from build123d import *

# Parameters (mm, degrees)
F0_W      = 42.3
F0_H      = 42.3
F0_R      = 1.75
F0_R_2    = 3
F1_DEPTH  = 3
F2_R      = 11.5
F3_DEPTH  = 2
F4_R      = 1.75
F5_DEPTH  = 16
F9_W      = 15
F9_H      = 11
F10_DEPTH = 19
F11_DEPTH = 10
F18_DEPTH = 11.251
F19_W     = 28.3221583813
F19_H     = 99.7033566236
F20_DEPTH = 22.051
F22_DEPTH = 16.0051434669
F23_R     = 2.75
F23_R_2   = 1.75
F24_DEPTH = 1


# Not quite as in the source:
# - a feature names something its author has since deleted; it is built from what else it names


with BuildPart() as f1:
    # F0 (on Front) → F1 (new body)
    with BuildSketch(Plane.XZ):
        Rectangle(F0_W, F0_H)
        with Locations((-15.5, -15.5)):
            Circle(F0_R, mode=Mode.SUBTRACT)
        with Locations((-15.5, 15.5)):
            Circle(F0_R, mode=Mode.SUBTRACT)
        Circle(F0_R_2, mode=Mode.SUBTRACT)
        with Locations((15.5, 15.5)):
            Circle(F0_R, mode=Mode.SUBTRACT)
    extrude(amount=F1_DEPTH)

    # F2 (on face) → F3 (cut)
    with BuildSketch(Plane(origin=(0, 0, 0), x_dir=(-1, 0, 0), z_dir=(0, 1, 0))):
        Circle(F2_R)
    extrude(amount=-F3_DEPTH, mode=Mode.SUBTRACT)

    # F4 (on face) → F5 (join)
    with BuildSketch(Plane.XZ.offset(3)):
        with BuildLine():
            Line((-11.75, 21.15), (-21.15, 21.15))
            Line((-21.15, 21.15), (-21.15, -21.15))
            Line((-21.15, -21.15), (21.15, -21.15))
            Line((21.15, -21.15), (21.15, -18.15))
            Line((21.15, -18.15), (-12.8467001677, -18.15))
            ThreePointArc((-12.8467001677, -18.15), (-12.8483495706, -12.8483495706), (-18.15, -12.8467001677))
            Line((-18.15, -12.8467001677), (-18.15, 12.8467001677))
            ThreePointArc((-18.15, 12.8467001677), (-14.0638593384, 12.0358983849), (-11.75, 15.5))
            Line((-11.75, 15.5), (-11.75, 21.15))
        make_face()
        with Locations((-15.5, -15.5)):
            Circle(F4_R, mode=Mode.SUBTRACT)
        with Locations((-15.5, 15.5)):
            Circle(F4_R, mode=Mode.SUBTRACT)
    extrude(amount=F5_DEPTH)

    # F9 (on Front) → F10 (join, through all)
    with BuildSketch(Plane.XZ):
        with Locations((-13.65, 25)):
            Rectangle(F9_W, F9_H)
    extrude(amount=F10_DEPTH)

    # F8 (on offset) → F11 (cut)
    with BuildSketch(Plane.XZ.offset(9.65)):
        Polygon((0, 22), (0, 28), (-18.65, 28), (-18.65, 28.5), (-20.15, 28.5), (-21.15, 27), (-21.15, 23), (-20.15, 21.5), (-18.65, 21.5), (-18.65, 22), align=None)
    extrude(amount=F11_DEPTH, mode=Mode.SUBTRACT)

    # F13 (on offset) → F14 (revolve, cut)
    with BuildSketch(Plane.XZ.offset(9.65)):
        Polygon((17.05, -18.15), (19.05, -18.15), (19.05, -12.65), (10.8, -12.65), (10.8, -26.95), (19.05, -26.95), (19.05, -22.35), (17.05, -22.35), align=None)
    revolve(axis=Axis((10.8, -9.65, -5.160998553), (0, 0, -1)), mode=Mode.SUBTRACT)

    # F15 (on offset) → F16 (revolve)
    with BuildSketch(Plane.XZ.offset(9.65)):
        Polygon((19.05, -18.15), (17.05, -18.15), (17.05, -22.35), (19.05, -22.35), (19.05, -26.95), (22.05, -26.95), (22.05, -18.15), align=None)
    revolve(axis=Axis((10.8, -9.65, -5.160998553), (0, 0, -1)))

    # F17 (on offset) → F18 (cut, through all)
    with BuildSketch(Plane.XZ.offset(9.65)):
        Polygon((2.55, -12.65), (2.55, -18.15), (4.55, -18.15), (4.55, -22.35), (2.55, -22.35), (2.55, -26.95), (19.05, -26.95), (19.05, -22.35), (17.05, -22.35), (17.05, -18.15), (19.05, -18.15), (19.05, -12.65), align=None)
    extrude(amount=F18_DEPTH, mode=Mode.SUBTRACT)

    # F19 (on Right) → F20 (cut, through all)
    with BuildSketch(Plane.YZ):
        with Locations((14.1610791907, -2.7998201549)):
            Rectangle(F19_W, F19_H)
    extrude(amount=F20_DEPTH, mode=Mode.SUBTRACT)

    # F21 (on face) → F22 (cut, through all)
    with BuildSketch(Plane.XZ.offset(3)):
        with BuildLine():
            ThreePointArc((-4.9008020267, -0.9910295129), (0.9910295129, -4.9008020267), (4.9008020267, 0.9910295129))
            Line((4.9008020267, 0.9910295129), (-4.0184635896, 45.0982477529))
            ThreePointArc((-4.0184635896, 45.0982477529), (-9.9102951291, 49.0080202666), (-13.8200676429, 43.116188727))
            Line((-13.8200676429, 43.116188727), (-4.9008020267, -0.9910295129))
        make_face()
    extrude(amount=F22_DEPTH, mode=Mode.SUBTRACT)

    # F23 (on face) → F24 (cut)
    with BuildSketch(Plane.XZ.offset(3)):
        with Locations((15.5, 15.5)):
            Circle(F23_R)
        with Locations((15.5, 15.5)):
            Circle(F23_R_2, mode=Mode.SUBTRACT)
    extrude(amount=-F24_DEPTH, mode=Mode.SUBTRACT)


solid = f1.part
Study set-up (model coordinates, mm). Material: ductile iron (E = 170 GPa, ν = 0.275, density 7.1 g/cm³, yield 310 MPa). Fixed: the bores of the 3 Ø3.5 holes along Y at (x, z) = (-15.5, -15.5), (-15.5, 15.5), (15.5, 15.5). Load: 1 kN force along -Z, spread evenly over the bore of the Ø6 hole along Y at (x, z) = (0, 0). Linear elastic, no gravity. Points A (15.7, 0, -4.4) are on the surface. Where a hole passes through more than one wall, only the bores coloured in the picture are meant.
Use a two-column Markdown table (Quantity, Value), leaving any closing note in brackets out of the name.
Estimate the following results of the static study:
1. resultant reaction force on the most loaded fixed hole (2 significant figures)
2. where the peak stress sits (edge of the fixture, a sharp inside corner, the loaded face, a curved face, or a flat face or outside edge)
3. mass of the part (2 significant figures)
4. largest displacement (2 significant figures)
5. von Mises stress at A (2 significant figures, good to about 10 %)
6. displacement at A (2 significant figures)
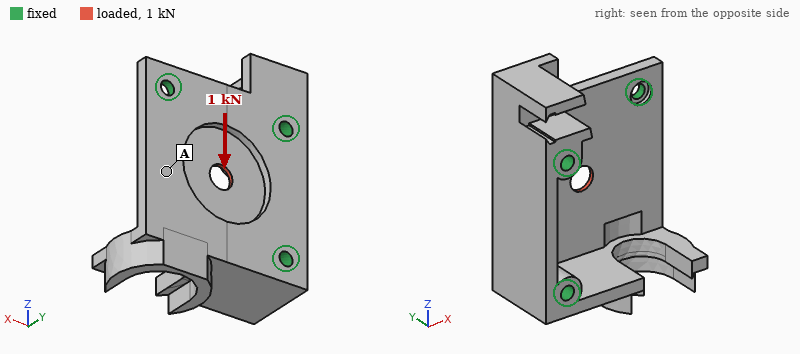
| Quantity | Value |
|---|---|
| resultant reaction force on the most loaded fixed hole | 400 N |
| where the peak stress sits | the loaded face |
| mass of the part | 79 g |
| largest displacement | 3.9 µm |
| von Mises stress at A | 7.1 MPa |
| displacement at A | 1.7 µm |
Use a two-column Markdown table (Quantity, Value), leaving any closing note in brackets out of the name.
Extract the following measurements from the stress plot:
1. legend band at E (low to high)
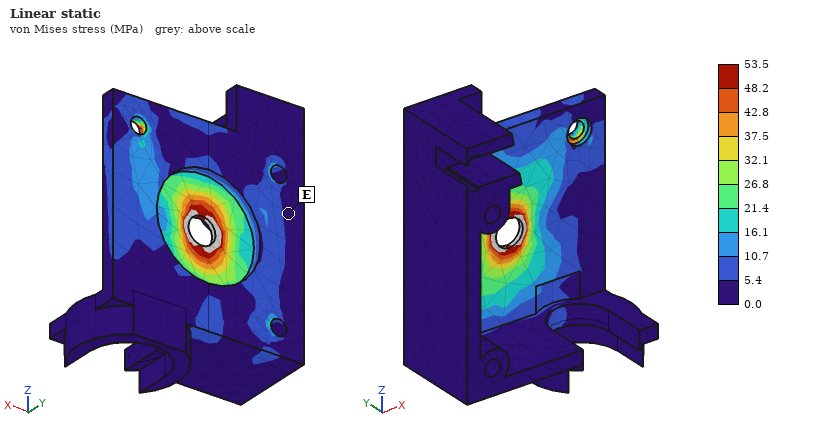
| Quantity | Value |
|---|---|
| legend band at E | 0.0 to 5.4 MPa |
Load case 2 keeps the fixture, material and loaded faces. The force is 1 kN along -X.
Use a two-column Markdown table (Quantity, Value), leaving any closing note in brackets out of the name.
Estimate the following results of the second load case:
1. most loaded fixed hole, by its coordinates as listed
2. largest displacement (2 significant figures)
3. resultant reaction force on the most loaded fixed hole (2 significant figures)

| Quantity | Value |
|---|---|
| most loaded fixed hole, by its coordinates as listed | (-15.5, -15.5) |
| largest displacement | 3.8 µm |
| resultant reaction force on the most loaded fixed hole | 450 N |
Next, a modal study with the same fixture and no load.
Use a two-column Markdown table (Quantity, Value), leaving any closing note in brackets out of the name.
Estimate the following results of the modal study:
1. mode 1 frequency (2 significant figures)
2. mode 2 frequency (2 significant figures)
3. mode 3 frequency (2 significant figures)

| Quantity | Value |
|---|---|
| mode 1 frequency | 4200 Hz |
| mode 2 frequency | 6100 Hz |
| mode 3 frequency | 9500 Hz |
